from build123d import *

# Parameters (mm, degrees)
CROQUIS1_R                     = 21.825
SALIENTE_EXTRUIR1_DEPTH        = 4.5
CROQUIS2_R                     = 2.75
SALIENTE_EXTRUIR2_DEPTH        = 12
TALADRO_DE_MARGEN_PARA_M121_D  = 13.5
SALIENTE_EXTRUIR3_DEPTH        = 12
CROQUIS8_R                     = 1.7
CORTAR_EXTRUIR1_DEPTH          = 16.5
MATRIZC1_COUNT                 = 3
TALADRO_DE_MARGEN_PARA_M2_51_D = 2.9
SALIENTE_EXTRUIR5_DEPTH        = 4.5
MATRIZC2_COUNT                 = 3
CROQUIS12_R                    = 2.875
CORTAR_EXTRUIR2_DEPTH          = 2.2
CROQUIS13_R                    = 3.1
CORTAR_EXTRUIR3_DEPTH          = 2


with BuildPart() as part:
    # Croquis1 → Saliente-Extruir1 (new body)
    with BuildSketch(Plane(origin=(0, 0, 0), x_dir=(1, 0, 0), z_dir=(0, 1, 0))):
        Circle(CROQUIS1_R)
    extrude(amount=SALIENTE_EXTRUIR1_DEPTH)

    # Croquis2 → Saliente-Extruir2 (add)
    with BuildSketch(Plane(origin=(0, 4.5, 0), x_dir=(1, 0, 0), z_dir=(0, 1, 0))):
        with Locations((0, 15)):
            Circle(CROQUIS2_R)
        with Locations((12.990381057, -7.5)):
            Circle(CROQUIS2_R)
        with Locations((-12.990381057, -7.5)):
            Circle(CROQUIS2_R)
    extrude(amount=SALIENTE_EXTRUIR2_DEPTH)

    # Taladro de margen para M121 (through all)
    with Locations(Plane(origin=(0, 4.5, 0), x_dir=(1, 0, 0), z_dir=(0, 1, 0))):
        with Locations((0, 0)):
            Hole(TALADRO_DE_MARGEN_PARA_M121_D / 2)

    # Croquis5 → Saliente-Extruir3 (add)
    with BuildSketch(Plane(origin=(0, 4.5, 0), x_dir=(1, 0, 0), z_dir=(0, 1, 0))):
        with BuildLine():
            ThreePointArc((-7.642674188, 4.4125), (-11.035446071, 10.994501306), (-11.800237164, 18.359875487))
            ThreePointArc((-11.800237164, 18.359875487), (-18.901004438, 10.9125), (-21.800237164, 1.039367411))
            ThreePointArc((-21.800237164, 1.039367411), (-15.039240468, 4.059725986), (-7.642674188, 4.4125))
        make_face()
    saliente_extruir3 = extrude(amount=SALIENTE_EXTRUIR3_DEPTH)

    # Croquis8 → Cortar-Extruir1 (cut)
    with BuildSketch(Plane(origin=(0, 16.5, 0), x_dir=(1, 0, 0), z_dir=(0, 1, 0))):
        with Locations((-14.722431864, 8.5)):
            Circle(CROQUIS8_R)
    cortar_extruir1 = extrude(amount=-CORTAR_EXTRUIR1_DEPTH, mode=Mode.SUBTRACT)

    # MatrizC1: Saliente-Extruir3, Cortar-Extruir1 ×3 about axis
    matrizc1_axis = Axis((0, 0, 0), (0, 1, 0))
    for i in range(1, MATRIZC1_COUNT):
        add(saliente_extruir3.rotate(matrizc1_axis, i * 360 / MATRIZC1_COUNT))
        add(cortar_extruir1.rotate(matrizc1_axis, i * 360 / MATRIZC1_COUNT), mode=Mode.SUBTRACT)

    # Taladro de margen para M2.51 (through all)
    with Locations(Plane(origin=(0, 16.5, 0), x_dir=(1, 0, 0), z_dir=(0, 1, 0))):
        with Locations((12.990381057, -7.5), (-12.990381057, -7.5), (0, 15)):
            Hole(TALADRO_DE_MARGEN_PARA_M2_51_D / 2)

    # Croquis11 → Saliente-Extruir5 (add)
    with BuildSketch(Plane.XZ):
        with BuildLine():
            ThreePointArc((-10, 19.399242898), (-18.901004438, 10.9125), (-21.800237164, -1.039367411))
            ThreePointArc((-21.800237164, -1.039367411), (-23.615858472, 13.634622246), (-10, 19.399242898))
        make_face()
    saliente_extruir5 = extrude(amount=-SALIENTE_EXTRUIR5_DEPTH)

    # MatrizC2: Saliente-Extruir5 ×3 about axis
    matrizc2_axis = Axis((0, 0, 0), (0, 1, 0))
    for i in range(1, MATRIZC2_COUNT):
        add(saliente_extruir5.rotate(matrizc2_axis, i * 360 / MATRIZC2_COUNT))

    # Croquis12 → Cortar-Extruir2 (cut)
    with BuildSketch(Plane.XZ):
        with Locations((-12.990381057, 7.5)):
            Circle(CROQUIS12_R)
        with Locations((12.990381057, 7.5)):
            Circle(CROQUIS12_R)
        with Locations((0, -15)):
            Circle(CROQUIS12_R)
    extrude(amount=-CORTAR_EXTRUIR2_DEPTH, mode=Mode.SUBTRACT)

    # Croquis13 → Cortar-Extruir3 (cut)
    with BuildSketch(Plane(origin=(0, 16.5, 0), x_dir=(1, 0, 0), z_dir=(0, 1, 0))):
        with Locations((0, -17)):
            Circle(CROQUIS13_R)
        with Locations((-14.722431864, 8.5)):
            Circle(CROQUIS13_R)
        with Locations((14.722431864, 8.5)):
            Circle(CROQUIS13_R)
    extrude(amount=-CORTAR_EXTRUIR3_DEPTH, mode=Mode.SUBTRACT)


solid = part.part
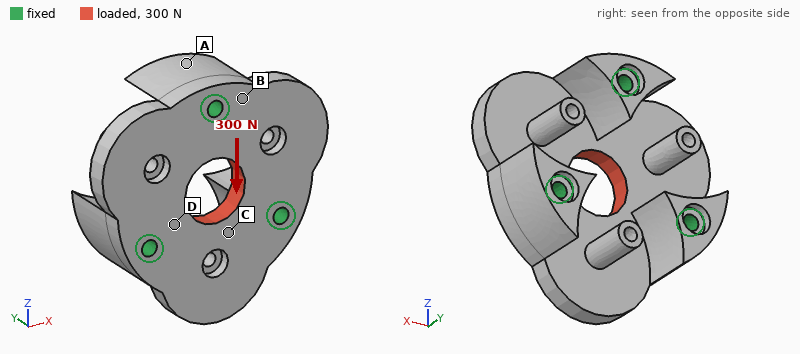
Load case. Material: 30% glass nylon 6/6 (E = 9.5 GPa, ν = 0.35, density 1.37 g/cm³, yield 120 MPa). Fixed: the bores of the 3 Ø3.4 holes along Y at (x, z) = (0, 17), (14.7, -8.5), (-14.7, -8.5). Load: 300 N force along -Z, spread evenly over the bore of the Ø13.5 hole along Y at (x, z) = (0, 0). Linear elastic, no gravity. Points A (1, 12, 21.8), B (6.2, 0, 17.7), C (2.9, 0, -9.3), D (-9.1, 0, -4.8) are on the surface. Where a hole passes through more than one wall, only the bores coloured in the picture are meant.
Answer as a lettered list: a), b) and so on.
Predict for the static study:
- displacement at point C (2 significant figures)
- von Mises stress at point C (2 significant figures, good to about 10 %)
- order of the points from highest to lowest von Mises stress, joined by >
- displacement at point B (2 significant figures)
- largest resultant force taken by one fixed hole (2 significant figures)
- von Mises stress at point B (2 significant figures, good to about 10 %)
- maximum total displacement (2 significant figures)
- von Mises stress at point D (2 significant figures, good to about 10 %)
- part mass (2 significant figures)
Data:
a) 3.7 µm
b) 1.6 MPa
c) C > D > B > A
d) 1.0 µm
e) 100 N
f) 0.77 MPa
g) 4.5 µm
h) 1.3 MPa
i) 15 g
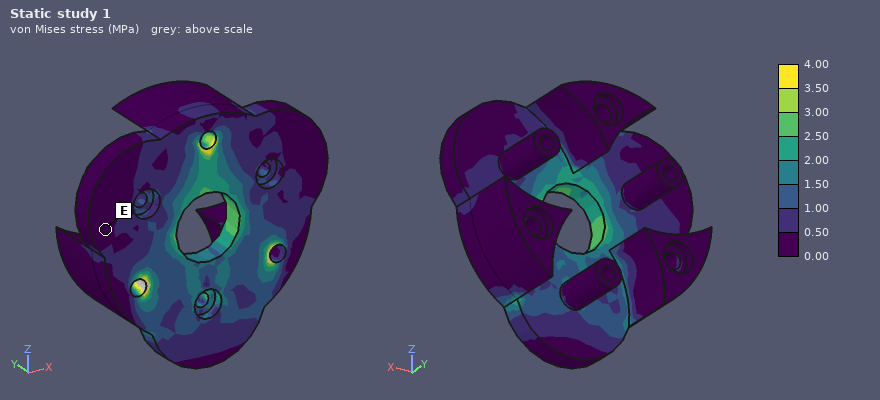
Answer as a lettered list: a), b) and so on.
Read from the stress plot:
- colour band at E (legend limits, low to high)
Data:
a) 0.00 to 0.50 MPa
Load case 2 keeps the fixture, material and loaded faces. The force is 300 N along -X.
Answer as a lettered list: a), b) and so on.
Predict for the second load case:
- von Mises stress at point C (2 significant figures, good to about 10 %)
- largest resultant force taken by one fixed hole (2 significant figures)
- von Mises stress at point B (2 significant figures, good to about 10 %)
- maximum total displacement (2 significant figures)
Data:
a) 1.1 MPa
b) 100 N
c) 1.2 MPa
d) 4.0 µm
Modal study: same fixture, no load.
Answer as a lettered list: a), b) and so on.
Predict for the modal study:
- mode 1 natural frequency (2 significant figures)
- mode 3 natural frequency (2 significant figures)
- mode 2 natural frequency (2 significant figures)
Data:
a) 7100 Hz
b) 7200 Hz
c) 7100 Hz
